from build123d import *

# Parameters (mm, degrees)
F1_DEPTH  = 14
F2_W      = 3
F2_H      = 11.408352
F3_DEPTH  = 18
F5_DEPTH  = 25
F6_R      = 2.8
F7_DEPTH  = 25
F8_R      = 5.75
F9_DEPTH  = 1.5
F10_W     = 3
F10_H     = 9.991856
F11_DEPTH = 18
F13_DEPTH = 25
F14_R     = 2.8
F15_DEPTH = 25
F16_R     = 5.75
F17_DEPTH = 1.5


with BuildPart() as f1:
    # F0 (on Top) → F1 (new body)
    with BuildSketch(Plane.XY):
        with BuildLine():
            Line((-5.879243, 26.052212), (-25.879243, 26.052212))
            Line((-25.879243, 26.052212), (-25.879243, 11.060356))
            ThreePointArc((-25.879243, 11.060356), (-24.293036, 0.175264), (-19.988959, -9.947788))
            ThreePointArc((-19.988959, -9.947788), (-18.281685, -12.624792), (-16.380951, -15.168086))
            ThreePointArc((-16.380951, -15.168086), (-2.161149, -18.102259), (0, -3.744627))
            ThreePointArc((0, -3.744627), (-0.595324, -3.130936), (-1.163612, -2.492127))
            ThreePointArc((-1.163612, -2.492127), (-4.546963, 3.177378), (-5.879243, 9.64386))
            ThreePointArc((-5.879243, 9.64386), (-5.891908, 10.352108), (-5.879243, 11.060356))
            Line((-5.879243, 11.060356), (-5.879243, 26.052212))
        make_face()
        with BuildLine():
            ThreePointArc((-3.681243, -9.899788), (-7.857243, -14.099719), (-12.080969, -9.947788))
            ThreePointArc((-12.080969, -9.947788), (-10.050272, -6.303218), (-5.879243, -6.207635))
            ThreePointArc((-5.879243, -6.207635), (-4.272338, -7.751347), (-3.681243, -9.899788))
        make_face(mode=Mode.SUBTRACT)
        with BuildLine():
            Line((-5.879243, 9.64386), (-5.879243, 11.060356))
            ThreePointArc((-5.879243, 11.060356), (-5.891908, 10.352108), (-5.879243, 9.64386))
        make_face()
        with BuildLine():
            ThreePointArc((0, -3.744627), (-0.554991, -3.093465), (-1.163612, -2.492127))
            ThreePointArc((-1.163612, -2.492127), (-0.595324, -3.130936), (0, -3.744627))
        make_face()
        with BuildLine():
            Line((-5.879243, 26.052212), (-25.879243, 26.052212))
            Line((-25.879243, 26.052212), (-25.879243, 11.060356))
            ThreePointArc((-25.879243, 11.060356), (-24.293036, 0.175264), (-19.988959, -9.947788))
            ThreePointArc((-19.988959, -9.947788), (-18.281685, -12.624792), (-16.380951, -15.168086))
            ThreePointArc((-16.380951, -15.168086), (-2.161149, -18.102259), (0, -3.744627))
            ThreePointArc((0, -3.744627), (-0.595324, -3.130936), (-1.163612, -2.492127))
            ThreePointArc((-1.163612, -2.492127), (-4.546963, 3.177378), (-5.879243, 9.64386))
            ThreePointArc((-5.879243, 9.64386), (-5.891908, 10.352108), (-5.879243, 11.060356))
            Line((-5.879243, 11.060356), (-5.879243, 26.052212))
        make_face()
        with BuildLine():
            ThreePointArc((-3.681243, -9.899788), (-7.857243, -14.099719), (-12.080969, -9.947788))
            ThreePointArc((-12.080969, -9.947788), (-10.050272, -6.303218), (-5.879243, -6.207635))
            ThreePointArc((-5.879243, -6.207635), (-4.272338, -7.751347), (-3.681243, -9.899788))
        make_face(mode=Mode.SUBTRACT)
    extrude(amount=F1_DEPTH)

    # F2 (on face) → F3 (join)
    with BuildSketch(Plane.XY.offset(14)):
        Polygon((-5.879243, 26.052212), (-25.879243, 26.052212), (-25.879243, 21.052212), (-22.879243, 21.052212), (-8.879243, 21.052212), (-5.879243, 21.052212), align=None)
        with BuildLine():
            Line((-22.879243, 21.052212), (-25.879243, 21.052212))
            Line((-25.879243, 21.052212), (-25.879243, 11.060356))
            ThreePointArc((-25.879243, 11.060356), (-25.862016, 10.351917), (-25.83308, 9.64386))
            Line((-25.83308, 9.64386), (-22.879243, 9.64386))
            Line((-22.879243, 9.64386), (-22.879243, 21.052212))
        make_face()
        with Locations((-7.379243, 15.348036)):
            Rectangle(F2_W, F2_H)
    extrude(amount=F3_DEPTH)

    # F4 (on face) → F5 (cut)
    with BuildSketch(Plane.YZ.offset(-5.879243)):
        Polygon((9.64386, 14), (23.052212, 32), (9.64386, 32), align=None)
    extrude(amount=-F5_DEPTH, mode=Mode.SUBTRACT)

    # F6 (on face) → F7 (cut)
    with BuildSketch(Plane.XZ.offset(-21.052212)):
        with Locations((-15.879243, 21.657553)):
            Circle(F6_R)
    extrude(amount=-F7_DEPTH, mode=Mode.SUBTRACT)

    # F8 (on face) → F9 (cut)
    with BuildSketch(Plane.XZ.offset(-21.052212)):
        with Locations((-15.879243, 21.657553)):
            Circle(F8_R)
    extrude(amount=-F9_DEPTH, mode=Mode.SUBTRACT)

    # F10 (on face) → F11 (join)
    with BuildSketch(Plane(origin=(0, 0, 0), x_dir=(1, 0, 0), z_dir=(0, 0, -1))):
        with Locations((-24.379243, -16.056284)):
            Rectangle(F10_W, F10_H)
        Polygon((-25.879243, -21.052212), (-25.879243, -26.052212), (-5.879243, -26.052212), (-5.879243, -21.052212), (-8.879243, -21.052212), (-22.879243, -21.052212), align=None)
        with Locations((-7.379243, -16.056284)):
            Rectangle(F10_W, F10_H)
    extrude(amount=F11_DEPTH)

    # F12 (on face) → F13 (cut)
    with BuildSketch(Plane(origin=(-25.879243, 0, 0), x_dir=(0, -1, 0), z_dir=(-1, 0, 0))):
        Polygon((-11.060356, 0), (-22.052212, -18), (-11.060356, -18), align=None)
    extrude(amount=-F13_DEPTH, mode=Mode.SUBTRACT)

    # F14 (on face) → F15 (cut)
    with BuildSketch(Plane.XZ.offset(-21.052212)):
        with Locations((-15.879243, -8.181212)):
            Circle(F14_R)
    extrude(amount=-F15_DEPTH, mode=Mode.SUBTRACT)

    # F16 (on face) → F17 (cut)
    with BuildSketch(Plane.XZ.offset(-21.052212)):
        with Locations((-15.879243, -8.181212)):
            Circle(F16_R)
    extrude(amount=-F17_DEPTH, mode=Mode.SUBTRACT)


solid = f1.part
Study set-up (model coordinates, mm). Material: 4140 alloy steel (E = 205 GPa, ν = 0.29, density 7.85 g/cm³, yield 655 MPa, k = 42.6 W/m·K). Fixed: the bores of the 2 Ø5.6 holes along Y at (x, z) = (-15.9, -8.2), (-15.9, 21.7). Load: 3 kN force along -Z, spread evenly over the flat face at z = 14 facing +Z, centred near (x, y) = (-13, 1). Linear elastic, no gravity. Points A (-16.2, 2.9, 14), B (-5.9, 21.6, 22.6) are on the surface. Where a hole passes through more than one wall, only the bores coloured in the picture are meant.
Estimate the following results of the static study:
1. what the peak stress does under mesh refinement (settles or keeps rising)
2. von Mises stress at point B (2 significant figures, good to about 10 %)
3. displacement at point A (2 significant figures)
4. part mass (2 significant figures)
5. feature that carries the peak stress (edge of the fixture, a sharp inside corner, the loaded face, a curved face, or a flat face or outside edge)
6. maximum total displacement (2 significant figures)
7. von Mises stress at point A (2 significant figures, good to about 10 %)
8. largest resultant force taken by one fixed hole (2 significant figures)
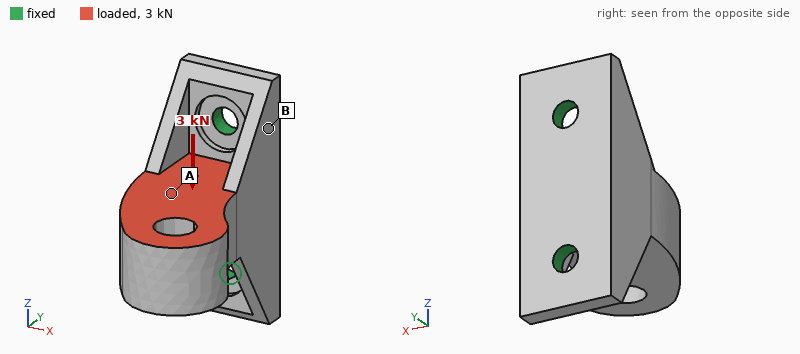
keeps rising
14 MPa
17 µm
130 g
edge of the fixture
44 µm
28 MPa
2.9 kN
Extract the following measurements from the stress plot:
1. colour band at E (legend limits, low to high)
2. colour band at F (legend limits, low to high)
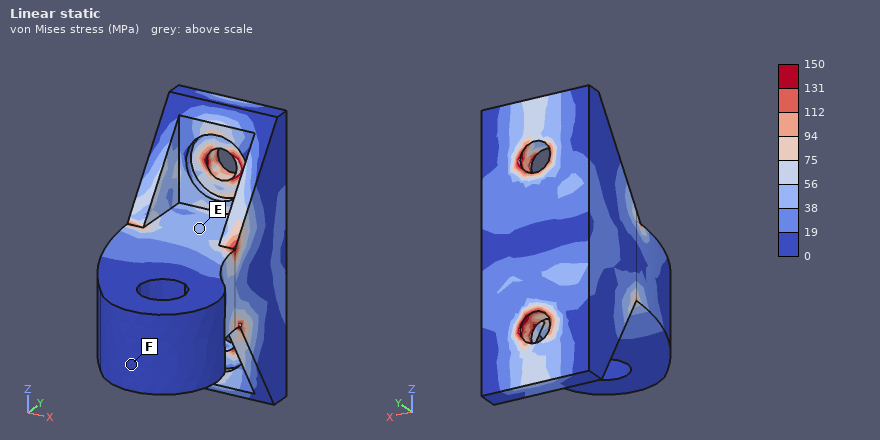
38 to 56 MPa
0 to 19 MPa
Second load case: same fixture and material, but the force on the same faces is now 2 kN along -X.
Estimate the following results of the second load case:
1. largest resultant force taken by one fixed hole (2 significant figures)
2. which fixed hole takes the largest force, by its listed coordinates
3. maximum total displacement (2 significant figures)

1.5 kN
(-15.9, 21.7)
0.12 mm
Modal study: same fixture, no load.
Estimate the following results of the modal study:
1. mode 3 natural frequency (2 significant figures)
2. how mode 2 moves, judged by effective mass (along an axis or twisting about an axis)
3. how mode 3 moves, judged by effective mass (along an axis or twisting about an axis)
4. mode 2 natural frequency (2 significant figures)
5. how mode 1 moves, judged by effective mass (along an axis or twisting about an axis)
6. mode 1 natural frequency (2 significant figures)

13 kHz
along Z
along Y
6000 Hz
along X
2800 Hz
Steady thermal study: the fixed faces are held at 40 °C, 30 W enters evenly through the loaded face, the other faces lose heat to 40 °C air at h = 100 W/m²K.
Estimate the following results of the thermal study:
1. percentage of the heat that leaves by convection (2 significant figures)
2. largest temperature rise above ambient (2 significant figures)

44 %
54 K
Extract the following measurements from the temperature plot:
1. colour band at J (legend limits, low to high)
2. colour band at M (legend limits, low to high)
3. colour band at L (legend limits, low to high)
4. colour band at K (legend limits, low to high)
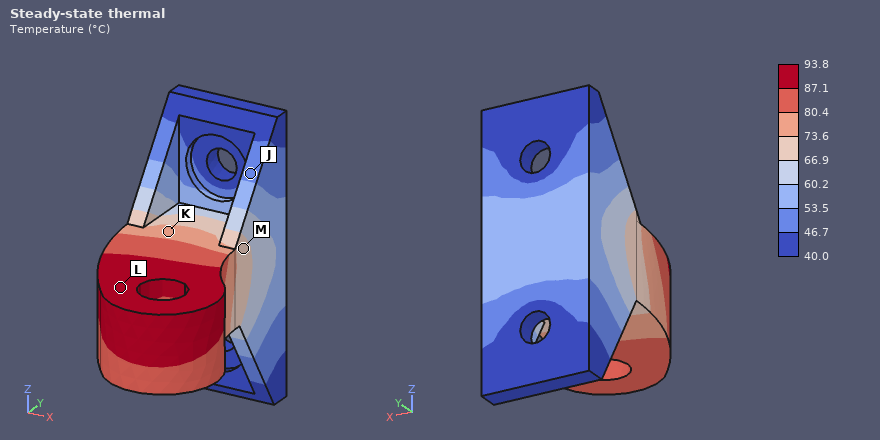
46.7 to 53.5 °C
66.9 to 73.6 °C
87.1 to 93.8 °C
73.6 to 80.4 °C
